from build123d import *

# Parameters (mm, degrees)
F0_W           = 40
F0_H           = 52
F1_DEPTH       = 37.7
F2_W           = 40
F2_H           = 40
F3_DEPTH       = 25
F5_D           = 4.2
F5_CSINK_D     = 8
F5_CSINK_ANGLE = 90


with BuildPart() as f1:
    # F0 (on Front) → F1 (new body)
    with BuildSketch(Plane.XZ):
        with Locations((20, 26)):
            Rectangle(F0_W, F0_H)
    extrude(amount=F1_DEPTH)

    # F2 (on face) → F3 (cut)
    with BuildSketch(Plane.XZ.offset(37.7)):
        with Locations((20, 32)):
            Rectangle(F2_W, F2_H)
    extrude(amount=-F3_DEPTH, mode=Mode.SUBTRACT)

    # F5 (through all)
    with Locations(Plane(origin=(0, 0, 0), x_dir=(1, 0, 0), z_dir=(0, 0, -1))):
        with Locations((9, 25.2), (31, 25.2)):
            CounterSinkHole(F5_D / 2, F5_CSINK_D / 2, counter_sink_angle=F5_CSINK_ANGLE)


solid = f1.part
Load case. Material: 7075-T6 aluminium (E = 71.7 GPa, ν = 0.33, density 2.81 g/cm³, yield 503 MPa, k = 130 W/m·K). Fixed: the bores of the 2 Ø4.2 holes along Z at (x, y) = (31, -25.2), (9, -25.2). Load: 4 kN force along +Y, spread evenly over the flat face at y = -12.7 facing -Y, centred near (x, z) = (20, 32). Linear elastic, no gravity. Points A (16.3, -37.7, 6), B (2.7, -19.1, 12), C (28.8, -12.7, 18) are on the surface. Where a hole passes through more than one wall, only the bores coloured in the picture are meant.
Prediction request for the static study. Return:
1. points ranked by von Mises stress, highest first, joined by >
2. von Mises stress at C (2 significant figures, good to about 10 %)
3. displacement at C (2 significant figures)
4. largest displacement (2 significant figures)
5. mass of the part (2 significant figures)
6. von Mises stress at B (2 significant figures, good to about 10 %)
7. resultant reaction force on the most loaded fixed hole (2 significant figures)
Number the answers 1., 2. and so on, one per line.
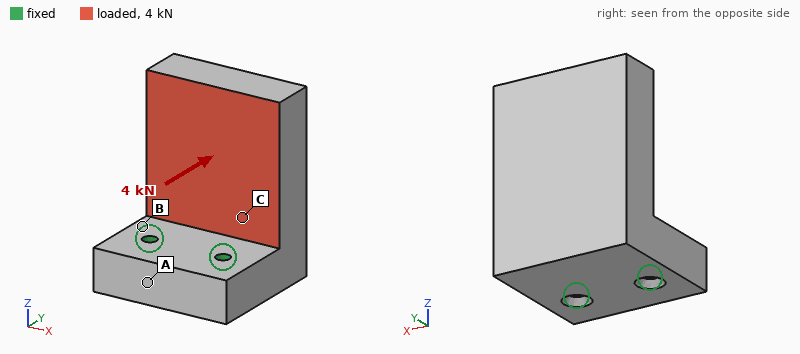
1. B > C > A
2. 50 MPa
3. 0.070 mm
4. 0.34 mm
5. 110 g
6. 95 MPa
7. 2.1 kN
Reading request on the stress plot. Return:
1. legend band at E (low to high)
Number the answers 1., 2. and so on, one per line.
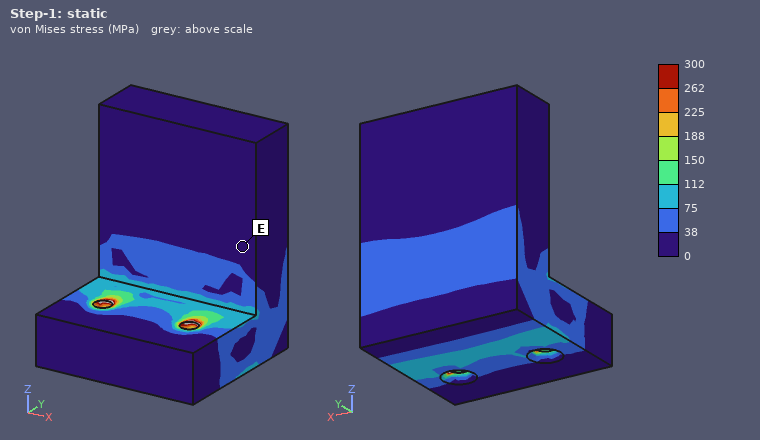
1. 0 to 38 MPa
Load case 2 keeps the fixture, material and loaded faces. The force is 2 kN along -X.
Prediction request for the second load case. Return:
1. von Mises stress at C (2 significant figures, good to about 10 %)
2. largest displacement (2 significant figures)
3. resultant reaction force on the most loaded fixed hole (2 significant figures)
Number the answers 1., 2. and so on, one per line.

1. 24 MPa
2. 67 µm
3. 2.2 kN
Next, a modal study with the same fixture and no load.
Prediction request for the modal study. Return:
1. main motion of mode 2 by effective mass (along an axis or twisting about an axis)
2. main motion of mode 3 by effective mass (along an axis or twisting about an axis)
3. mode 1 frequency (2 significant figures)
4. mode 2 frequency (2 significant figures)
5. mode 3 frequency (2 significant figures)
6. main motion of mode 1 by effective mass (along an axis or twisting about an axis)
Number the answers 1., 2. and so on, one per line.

1. along X
2. along Z
3. 2700 Hz
4. 4500 Hz
5. 8800 Hz
6. along Y
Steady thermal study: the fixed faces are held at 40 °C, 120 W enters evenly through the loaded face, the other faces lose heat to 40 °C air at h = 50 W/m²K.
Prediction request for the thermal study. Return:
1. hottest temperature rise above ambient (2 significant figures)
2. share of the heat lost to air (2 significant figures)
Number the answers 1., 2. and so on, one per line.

1. 71 K
2. 10 %
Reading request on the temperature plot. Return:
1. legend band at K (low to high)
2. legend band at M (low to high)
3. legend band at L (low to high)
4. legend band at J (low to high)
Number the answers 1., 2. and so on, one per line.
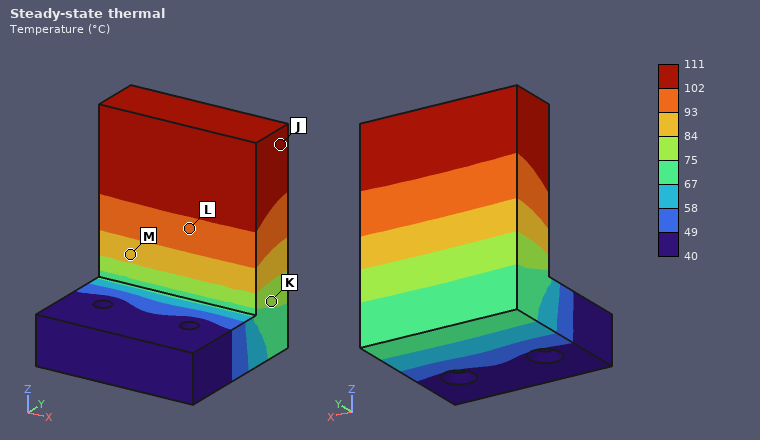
1. 75 to 84 °C
2. 84 to 93 °C
3. 93 to 102 °C
4. 102 to 111 °C
